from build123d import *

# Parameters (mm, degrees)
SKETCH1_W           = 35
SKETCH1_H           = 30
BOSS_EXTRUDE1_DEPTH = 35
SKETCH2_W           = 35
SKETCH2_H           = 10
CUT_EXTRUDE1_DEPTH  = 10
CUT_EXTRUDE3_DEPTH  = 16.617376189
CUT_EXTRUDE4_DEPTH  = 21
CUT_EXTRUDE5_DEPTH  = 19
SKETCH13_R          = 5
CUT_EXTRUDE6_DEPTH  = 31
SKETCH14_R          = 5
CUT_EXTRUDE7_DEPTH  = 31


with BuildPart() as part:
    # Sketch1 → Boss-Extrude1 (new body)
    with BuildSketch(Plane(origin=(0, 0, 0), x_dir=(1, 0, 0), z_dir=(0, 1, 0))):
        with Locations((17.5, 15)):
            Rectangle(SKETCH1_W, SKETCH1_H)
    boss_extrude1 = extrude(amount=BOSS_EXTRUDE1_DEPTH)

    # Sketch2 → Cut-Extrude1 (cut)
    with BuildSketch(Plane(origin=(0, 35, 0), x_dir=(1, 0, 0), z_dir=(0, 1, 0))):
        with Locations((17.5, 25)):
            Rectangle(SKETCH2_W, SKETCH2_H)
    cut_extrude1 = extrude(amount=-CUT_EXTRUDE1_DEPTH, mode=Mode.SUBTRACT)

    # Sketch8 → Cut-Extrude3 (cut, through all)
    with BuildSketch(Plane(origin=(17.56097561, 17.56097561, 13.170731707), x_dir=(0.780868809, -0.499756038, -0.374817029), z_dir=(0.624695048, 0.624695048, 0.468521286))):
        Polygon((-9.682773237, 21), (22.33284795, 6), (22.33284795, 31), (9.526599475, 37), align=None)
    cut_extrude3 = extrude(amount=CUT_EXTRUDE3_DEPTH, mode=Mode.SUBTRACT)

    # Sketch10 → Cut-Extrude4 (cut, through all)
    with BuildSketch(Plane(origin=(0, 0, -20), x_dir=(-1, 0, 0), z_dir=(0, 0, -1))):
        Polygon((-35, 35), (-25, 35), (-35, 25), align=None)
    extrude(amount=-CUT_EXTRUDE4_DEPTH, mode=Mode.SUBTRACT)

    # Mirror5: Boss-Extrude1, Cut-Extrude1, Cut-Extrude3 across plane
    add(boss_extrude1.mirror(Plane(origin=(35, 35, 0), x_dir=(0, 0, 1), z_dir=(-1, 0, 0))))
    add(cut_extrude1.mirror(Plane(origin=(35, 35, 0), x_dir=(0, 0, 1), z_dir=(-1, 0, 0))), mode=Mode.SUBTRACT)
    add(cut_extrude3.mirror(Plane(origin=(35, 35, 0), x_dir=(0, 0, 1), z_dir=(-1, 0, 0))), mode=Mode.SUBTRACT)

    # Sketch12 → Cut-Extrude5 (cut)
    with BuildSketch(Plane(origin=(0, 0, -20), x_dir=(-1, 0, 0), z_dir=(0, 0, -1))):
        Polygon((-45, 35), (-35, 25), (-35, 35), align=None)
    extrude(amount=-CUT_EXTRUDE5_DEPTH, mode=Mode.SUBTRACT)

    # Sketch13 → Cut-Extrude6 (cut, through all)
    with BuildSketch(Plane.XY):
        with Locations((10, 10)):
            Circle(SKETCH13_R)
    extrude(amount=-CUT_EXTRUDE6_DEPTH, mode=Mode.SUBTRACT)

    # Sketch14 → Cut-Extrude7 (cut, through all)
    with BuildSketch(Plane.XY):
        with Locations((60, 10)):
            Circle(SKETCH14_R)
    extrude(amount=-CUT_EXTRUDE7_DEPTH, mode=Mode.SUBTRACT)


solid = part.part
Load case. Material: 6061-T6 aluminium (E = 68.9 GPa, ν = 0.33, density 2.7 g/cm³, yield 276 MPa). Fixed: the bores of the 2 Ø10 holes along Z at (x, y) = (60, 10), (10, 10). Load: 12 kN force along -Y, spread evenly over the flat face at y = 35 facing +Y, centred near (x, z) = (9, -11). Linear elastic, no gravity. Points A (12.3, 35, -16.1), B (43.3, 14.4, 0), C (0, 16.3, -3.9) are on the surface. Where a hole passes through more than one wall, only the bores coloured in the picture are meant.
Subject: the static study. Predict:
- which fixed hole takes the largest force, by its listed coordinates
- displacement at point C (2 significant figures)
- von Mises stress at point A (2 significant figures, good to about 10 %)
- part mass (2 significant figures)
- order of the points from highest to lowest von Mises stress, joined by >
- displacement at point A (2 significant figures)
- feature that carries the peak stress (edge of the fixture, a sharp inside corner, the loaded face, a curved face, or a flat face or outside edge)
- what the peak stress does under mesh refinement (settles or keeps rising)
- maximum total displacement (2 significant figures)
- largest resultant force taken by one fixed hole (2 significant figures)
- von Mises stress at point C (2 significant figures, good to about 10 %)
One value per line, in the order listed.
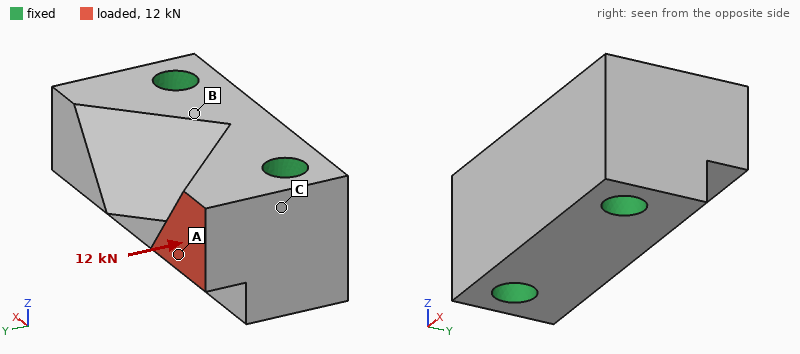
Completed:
(10, 10)
4.4 µm
32 MPa
150 g
A > C > B
10 µm
edge of the fixture
keeps rising
15 µm
12 kN
25 MPa
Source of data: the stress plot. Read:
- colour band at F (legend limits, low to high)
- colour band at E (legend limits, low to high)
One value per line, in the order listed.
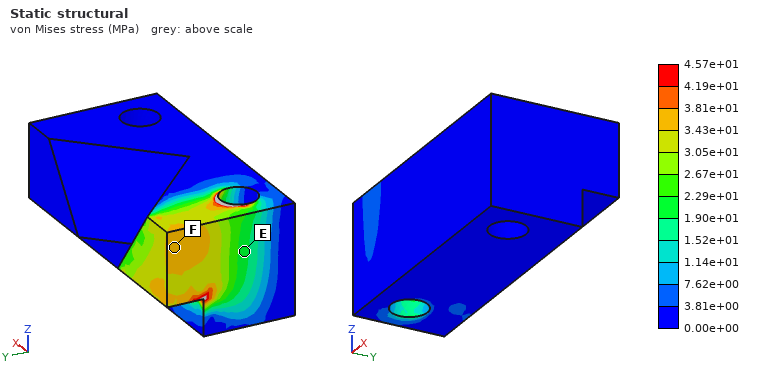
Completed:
3.43e+01 to 3.81e+01 MPa
1.90e+01 to 2.29e+01 MPa
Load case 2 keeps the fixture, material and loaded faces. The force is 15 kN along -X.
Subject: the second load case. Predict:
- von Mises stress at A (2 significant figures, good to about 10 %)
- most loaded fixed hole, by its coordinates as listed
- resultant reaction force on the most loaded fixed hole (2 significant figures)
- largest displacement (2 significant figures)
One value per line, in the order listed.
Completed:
93 MPa
(10, 10)
12 kN
67 µm
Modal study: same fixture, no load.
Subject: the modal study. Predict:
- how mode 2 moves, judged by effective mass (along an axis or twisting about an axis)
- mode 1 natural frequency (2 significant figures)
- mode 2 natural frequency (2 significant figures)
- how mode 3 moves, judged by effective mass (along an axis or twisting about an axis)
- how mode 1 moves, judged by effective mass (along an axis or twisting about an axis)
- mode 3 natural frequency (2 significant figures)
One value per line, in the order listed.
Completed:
along Z
22 kHz
26 kHz
along X
along Y
30 kHz
